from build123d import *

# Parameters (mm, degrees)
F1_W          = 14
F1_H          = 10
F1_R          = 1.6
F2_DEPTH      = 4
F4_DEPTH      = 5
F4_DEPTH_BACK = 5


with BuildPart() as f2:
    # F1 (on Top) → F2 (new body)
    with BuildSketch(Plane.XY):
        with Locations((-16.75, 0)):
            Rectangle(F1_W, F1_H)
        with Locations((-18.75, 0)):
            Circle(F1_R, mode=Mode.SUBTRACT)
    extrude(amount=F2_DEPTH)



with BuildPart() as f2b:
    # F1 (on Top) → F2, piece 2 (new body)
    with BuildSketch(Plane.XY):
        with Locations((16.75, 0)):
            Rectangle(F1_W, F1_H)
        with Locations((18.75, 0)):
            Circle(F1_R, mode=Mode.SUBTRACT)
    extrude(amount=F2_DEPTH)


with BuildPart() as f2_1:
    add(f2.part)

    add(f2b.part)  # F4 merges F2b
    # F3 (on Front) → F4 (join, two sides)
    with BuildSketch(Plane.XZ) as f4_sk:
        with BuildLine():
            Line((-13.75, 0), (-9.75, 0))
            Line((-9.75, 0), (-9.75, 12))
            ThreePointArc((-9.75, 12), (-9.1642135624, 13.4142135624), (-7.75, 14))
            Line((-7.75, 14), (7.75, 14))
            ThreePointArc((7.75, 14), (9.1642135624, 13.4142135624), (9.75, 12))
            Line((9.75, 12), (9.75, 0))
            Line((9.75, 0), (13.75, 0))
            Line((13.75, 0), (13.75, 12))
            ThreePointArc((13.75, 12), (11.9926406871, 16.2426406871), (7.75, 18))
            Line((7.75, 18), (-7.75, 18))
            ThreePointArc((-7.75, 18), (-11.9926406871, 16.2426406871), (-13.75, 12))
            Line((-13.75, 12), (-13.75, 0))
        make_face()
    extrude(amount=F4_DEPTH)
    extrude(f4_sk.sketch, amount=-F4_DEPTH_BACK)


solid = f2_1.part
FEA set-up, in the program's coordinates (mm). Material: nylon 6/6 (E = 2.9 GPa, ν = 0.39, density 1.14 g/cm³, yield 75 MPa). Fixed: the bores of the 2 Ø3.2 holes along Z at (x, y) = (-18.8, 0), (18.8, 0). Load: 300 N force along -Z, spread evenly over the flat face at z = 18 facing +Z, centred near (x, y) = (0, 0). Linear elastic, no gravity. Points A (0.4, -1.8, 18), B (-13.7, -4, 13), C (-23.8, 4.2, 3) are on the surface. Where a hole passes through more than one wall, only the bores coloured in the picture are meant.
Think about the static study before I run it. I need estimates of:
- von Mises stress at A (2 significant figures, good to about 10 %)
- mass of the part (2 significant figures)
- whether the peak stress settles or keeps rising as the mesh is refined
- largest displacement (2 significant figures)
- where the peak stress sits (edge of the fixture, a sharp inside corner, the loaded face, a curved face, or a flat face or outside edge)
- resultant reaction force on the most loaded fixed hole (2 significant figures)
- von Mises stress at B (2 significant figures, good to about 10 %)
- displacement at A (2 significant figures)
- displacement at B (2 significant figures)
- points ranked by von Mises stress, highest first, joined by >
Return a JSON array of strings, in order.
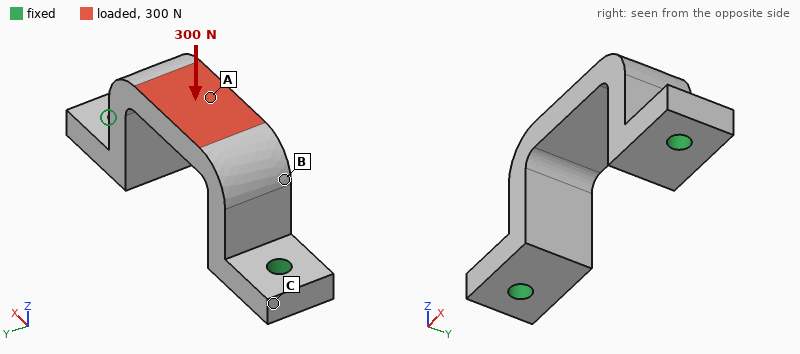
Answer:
["18 MPa", "3.2 g", "keeps rising", "0.20 mm", "edge of the fixture", "170 N", "8.1 MPa", "0.19 mm", "0.051 mm", "A > B > C"]
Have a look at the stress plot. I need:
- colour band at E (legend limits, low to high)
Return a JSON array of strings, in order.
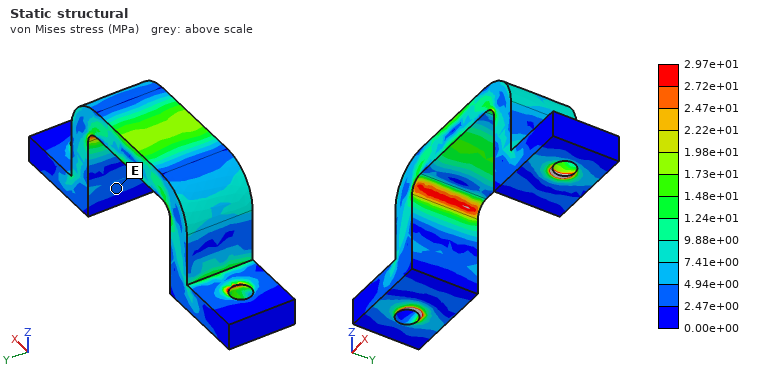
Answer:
["2.47e+00 to 4.94e+00 MPa"]
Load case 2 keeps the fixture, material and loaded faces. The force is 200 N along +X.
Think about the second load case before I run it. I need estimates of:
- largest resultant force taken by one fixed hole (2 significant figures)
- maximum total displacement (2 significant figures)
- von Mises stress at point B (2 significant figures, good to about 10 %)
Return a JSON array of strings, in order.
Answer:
["130 N", "0.29 mm", "9.8 MPa"]
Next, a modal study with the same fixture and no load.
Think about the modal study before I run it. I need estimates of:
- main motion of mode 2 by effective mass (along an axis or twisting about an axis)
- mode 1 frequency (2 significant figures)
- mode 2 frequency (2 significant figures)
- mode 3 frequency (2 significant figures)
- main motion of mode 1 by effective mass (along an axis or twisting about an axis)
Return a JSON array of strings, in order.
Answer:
["along X", "2300 Hz", "3400 Hz", "4600 Hz", "along Y"]
